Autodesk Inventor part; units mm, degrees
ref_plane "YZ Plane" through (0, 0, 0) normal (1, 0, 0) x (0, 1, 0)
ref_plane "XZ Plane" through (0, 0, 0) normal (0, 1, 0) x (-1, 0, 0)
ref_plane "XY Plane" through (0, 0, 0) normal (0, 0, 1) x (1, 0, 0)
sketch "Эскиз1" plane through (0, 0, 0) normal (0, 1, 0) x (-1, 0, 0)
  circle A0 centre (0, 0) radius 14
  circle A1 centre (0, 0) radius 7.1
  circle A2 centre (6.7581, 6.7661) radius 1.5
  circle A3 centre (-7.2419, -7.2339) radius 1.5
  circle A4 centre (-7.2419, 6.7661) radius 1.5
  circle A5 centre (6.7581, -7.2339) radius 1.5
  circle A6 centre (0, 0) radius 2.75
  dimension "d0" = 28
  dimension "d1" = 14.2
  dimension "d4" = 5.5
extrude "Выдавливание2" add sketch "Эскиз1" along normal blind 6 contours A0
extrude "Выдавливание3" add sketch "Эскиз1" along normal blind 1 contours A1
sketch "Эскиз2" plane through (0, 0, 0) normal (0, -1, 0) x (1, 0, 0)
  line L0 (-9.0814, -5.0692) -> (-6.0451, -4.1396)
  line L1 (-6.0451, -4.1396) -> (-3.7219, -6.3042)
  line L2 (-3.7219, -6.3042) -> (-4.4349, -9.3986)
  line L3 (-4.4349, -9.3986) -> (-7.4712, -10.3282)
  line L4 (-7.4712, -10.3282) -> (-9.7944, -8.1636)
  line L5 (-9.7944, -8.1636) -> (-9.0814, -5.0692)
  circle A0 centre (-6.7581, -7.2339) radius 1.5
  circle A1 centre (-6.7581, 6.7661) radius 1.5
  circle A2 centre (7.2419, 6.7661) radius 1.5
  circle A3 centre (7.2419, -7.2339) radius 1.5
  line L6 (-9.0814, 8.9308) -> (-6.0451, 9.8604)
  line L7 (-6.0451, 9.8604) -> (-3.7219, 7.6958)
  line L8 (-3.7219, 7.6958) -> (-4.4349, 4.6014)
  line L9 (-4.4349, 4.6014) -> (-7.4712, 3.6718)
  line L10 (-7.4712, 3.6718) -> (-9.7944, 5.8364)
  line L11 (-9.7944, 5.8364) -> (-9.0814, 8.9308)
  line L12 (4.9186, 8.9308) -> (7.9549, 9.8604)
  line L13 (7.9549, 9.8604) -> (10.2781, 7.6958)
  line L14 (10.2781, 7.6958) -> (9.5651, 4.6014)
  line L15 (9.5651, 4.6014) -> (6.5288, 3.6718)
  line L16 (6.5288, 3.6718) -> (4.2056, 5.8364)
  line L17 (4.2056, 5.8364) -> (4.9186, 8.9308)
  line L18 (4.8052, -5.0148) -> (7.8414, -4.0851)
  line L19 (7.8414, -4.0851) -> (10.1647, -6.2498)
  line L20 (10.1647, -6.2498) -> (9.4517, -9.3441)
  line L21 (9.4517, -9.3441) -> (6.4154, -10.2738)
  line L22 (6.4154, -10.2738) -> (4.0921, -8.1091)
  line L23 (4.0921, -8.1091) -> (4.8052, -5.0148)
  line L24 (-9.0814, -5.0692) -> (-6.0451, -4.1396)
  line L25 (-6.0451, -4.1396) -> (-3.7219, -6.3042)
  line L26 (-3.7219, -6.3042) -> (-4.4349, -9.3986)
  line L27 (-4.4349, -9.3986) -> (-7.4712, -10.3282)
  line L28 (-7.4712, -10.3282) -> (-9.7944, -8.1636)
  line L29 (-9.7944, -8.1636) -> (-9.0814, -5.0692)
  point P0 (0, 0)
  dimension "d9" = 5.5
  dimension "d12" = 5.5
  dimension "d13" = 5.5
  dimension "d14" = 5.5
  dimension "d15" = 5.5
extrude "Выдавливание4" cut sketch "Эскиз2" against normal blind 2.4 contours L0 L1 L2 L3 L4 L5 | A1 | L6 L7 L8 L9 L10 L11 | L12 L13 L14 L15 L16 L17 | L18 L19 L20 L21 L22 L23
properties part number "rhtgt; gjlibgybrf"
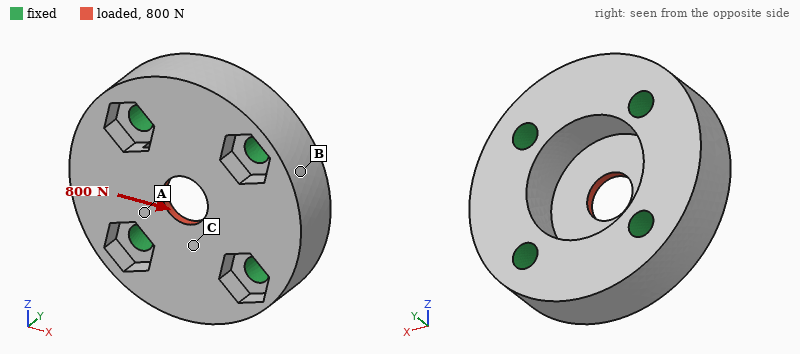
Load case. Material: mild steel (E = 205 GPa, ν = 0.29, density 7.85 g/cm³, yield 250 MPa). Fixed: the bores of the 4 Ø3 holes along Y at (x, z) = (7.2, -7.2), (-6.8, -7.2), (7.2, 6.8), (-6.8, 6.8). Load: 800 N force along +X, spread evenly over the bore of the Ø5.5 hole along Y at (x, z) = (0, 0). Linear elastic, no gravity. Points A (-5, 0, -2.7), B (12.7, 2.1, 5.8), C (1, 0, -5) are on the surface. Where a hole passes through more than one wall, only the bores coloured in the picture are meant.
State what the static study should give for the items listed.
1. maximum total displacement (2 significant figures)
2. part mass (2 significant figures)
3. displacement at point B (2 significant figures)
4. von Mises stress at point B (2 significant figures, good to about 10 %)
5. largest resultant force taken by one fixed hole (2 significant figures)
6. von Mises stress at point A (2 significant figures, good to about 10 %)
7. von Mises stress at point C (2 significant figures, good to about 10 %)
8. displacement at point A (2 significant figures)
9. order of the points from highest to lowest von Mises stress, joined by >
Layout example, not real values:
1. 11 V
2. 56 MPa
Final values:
1. 2.3 µm
2. 20 g
3. 0.74 µm
4. 9.7 MPa
5. 210 N
6. 39 MPa
7. 26 MPa
8. 1.5 µm
9. A > C > B
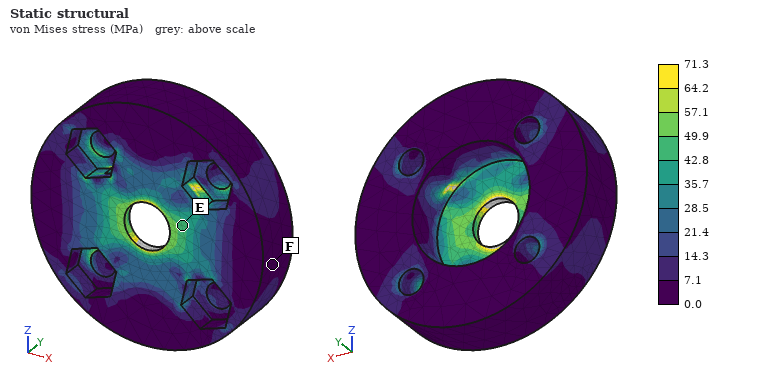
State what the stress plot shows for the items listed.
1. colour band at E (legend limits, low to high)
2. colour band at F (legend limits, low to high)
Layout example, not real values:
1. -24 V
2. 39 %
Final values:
1. 42.8 to 49.9 MPa
2. 0.0 to 7.1 MPa
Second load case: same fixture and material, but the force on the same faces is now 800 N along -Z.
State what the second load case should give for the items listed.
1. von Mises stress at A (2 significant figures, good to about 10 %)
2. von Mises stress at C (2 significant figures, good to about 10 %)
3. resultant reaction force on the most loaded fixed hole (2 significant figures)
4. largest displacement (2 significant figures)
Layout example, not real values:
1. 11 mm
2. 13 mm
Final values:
1. 26 MPa
2. 40 MPa
3. 210 N
4. 2.3 µm
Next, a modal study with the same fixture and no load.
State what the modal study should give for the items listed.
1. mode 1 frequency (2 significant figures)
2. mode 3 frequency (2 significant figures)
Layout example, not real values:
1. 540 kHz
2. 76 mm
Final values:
1. 45 kHz
2. 47 kHz
